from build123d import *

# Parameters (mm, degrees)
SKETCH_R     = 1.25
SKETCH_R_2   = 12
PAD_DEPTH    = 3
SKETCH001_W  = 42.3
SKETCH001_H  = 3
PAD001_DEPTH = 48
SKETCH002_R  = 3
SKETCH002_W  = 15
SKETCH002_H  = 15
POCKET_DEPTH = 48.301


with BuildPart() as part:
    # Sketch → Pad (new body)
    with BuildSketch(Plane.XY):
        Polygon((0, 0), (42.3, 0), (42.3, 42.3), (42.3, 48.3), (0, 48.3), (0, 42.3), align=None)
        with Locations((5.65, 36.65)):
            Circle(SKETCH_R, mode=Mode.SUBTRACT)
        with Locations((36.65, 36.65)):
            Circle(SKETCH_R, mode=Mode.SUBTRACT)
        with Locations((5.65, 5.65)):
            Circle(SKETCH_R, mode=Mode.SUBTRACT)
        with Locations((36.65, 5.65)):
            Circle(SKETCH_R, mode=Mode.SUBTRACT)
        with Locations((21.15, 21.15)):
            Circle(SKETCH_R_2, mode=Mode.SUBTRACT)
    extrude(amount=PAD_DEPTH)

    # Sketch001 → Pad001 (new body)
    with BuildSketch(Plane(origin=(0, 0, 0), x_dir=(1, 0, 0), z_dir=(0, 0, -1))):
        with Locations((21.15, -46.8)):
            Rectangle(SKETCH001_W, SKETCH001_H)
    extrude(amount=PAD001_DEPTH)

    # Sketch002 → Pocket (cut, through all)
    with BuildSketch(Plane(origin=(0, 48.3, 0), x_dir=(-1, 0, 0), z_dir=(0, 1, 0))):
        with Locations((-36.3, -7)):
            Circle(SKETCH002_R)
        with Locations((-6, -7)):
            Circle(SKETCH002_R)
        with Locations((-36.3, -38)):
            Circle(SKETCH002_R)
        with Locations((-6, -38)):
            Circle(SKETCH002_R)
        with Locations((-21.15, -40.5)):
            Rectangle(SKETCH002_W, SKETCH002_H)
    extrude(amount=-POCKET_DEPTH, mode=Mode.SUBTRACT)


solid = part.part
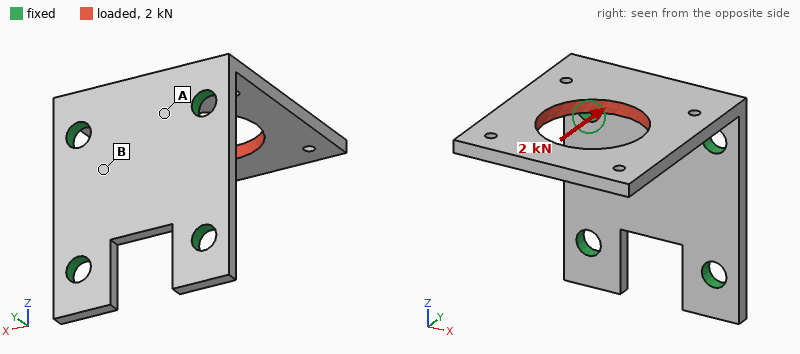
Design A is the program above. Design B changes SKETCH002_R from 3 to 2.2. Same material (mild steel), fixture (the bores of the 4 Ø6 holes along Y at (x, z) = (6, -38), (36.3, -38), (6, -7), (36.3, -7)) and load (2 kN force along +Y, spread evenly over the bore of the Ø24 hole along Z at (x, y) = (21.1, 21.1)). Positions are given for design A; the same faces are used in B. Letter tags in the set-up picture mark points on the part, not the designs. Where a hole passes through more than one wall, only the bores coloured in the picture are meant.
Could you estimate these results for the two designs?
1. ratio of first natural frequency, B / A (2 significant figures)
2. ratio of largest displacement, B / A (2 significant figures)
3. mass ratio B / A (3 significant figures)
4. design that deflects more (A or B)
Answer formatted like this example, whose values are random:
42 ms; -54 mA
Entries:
0.98; 1.3; 1.02; B
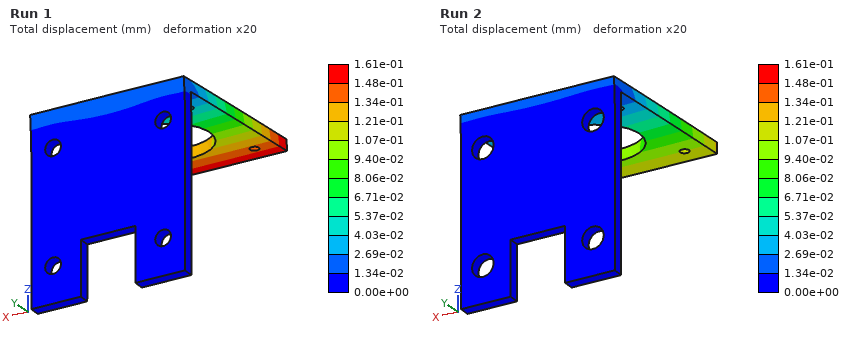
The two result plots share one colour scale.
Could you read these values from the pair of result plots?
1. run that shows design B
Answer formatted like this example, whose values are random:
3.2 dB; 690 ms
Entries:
Run 1
